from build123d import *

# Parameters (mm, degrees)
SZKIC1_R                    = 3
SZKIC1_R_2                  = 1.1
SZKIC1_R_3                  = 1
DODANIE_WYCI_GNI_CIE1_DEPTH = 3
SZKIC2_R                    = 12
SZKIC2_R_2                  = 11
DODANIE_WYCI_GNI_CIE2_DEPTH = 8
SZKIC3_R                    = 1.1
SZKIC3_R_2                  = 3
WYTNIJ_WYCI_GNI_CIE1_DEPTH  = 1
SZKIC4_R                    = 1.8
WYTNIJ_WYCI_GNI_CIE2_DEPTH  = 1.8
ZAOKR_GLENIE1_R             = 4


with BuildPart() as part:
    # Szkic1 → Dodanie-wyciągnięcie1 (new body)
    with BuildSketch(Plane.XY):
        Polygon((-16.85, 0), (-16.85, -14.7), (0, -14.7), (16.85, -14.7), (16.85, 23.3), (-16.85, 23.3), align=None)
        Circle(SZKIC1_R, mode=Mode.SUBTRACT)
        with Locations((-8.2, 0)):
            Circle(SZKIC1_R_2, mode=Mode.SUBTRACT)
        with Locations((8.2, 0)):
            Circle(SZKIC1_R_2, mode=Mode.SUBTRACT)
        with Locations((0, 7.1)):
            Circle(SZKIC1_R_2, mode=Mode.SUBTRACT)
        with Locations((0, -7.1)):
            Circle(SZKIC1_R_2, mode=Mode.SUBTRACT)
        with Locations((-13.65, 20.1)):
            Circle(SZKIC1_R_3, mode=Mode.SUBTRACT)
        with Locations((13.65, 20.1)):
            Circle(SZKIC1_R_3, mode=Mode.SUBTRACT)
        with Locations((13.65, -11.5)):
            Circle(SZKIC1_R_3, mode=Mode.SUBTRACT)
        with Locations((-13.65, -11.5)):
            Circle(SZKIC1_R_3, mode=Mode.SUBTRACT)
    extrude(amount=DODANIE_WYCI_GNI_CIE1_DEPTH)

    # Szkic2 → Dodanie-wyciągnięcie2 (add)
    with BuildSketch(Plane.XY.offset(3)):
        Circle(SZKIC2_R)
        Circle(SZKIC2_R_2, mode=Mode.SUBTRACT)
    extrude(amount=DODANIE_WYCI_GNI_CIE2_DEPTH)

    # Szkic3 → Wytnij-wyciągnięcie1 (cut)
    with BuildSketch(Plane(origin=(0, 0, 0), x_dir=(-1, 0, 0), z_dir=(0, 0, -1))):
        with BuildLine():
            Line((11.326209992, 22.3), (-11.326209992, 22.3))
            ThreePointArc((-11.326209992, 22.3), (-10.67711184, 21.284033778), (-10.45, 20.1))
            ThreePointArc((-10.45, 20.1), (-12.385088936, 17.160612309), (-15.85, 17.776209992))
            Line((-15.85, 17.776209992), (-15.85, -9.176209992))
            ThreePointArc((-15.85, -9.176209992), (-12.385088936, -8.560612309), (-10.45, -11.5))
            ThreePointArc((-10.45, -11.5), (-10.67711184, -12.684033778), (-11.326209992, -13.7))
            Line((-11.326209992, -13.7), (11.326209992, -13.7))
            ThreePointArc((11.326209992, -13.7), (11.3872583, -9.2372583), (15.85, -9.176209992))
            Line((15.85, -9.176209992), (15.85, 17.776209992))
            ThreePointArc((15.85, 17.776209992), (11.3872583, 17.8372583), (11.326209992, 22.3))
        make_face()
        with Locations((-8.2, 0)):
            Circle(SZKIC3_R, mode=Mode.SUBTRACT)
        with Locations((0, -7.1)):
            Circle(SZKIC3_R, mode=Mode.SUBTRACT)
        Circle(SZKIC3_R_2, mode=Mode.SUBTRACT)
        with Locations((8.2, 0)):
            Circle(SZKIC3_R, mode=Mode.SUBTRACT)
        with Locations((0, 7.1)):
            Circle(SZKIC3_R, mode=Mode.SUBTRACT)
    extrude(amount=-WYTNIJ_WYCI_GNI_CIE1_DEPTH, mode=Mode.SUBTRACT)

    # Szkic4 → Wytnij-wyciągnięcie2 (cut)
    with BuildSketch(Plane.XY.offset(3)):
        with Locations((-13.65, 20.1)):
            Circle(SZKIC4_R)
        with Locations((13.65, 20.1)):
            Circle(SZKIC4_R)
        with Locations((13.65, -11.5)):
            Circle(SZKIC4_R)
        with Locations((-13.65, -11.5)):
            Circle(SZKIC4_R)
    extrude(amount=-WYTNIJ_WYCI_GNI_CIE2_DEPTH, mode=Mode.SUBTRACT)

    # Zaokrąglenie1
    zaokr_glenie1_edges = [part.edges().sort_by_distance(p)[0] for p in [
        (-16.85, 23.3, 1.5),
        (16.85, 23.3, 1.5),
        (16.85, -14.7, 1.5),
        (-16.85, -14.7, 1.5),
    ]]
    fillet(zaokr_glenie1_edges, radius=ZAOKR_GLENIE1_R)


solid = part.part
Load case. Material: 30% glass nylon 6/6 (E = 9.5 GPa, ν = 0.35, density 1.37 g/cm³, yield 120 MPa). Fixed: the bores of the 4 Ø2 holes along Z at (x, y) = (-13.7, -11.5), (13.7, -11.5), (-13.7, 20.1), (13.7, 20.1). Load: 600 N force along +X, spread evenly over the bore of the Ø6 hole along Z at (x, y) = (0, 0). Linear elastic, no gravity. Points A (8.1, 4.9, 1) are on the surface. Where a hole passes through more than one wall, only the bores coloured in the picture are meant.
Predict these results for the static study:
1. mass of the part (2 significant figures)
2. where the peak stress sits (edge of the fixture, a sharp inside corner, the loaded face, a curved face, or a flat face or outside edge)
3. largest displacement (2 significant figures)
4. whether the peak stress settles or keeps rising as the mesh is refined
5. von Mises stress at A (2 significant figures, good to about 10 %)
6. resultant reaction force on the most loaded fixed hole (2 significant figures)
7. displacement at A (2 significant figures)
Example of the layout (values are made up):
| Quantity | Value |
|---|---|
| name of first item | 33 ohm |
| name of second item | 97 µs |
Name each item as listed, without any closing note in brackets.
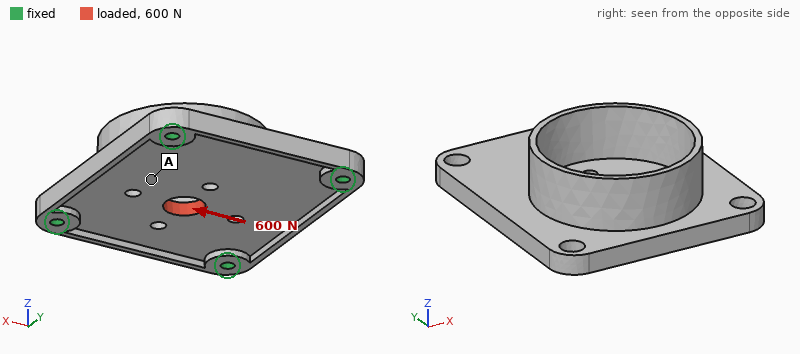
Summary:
| Quantity | Value |
|---|---|
| mass of the part | 4.3 g |
| where the peak stress sits | edge of the fixture |
| largest displacement | 40 µm |
| whether the peak stress settles or keeps rising as the mesh is refined | keeps rising |
| von Mises stress at A | 6.9 MPa |
| resultant reaction force on the most loaded fixed hole | 190 N |
| displacement at A | 32 µm |
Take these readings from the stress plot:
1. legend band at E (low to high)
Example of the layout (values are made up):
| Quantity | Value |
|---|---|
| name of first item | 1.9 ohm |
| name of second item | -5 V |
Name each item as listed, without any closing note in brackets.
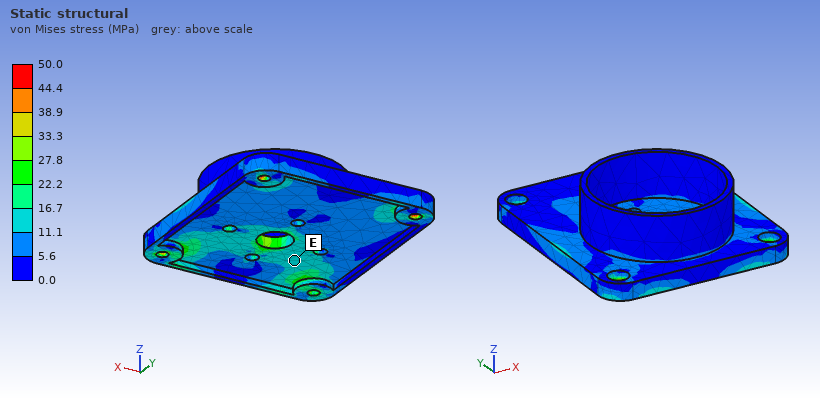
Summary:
| Quantity | Value |
|---|---|
| legend band at E | 11.1 to 16.7 MPa |
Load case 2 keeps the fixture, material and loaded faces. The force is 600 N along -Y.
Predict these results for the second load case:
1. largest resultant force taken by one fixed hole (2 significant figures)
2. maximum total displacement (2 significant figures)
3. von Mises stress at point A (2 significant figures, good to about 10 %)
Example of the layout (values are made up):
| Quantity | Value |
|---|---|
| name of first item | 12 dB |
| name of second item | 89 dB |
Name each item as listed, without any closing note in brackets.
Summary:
| Quantity | Value |
|---|---|
| largest resultant force taken by one fixed hole | 160 N |
| maximum total displacement | 39 µm |
| von Mises stress at point A | 7.5 MPa |
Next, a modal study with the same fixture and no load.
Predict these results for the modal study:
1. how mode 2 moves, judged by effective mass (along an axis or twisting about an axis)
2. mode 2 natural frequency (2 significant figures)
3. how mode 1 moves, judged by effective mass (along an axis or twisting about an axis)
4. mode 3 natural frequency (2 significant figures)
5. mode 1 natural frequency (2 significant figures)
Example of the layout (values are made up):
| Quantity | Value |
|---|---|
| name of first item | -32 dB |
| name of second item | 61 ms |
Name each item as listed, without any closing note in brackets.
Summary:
| Quantity | Value |
|---|---|
| how mode 2 moves, judged by effective mass | twisting about Y |
| mode 2 natural frequency | 6100 Hz |
| how mode 1 moves, judged by effective mass | along Z |
| mode 3 natural frequency | 6800 Hz |
| mode 1 natural frequency | 4400 Hz |
